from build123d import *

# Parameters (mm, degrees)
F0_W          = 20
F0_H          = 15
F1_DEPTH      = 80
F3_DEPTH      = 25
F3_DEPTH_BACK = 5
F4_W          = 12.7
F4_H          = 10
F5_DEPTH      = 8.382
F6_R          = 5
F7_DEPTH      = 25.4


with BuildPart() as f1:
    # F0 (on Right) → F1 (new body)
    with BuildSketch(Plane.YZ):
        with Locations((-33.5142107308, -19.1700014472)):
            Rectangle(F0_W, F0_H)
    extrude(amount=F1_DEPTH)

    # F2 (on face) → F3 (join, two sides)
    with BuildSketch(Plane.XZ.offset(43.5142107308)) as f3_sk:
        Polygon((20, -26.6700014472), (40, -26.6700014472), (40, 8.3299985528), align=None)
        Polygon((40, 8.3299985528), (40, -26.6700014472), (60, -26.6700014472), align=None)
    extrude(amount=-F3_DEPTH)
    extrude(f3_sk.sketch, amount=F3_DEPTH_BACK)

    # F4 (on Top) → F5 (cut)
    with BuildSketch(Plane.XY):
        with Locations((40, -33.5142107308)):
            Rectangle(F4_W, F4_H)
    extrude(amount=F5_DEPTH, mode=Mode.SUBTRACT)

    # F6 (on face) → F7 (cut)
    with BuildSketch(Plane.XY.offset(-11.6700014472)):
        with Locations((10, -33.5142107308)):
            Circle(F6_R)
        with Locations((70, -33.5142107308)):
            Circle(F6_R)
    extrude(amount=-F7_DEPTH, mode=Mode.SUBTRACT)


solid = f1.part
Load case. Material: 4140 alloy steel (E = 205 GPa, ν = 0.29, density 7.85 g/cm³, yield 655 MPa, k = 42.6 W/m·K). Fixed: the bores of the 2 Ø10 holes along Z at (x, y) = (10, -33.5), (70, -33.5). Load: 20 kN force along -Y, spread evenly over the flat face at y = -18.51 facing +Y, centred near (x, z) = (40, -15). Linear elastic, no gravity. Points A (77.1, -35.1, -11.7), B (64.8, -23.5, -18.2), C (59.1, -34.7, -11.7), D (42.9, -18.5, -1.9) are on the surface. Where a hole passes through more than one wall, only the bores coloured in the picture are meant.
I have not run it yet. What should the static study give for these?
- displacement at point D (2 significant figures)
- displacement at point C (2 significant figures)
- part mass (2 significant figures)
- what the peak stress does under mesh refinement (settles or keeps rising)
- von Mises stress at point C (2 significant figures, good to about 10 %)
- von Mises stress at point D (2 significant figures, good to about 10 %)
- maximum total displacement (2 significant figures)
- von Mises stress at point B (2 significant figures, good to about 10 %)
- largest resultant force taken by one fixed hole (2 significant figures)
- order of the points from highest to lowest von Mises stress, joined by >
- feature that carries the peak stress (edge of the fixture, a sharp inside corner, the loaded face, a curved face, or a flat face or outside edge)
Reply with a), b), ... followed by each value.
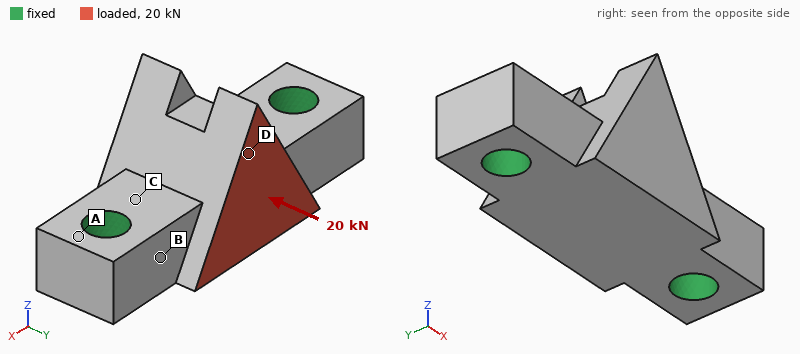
a) 32 µm
b) 7.8 µm
c) 260 g
d) keeps rising
e) 140 MPa
f) 38 MPa
g) 43 µm
h) 69 MPa
i) 10 kN
j) C > B > D > A
k) edge of the fixture
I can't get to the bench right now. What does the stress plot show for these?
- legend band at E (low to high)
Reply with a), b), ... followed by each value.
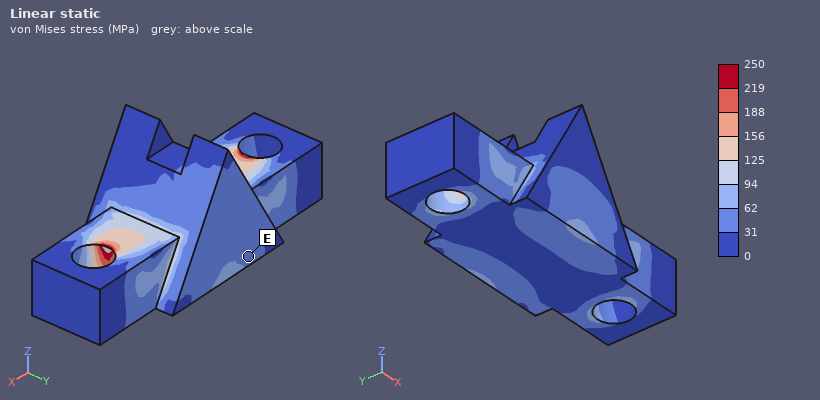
a) 31 to 62 MPa
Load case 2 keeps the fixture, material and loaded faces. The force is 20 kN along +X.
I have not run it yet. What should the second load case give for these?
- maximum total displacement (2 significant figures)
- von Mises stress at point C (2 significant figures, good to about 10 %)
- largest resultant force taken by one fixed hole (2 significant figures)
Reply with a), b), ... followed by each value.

a) 23 µm
b) 46 MPa
c) 12 kN
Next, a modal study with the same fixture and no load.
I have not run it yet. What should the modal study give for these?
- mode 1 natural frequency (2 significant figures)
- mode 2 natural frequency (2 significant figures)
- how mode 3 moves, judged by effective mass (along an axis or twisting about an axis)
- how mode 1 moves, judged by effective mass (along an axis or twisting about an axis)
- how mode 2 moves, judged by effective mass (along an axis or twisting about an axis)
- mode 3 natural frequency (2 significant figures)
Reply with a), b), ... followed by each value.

a) 11 kHz
b) 15 kHz
c) along Y
d) along Y
e) along Z
f) 18 kHz
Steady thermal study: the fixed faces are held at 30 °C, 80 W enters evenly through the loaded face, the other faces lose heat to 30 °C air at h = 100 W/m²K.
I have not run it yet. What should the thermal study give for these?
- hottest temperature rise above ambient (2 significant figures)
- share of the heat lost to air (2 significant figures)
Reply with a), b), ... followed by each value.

a) 81 K
b) 22 %
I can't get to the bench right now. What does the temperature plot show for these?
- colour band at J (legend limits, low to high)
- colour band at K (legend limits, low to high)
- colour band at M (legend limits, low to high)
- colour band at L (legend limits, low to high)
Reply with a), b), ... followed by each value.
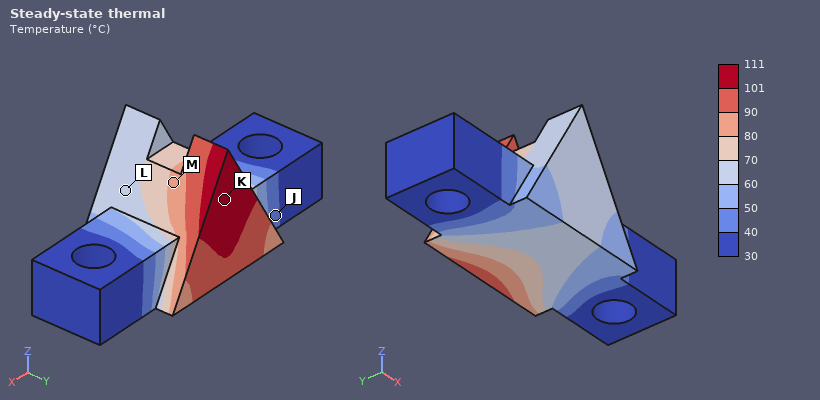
a) 40 to 50 °C
b) 101 to 111 °C
c) 80 to 90 °C
d) 60 to 70 °C
